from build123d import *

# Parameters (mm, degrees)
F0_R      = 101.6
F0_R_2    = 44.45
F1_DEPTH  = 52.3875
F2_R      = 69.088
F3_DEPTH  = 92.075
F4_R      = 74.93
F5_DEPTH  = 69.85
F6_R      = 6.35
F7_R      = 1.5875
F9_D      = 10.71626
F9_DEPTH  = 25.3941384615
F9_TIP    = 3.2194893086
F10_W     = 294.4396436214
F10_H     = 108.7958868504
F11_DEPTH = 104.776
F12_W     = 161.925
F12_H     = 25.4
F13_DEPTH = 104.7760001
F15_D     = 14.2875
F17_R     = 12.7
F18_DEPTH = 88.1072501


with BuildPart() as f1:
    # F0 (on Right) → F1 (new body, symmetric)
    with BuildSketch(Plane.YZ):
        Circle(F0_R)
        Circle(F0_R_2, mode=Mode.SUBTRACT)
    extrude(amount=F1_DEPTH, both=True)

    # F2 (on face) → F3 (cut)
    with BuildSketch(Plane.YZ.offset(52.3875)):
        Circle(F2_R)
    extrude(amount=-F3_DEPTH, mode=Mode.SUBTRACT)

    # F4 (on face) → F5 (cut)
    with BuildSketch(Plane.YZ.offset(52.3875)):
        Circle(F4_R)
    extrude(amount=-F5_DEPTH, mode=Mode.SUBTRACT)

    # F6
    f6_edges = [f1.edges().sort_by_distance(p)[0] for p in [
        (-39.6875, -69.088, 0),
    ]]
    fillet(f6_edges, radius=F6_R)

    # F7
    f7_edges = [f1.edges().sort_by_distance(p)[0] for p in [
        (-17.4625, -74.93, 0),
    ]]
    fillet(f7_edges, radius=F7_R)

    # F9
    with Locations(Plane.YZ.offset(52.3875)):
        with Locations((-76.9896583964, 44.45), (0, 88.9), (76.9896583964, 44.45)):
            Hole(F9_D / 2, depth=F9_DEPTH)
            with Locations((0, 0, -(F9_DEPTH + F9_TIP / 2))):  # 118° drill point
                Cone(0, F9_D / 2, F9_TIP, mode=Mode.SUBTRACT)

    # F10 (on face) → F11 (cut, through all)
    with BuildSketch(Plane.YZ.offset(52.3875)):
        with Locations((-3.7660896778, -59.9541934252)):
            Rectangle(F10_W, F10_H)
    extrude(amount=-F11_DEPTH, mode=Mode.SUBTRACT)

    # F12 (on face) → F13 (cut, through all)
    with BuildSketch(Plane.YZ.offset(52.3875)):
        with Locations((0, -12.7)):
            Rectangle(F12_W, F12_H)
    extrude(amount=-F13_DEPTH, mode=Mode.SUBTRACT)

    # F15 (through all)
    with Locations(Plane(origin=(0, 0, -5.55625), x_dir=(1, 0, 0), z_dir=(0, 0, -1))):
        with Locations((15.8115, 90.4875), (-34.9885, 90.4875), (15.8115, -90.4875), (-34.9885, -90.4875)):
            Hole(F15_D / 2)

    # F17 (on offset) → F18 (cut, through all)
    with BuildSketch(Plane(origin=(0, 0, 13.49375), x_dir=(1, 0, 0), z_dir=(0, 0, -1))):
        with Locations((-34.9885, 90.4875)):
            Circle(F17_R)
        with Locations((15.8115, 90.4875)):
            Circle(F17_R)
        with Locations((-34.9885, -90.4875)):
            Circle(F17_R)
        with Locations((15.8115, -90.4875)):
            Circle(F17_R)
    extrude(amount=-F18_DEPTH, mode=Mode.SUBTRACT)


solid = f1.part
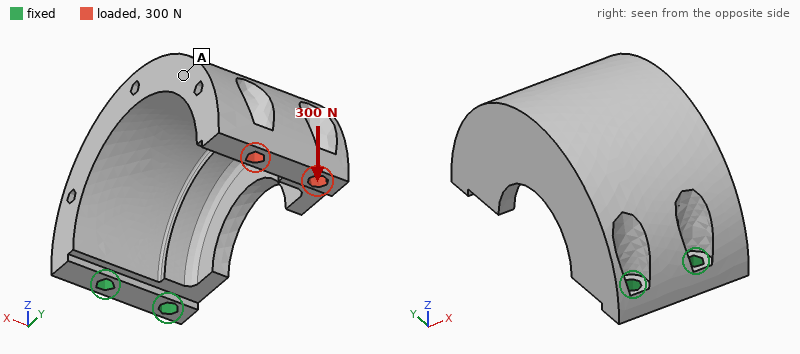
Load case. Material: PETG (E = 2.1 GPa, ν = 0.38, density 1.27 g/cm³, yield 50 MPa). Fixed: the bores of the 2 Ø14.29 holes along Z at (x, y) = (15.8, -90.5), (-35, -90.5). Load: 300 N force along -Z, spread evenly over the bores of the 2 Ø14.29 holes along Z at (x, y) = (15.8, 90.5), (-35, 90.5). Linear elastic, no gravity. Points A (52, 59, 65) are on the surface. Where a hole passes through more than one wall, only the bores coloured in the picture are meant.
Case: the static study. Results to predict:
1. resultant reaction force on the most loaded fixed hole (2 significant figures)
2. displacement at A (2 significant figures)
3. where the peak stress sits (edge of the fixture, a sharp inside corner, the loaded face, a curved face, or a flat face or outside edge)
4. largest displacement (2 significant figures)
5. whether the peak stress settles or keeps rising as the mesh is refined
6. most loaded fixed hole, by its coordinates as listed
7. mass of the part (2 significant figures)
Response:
230 N
2.0 mm
edge of the fixture
2.8 mm
keeps rising
(-35, -90.5)
1.0 kg
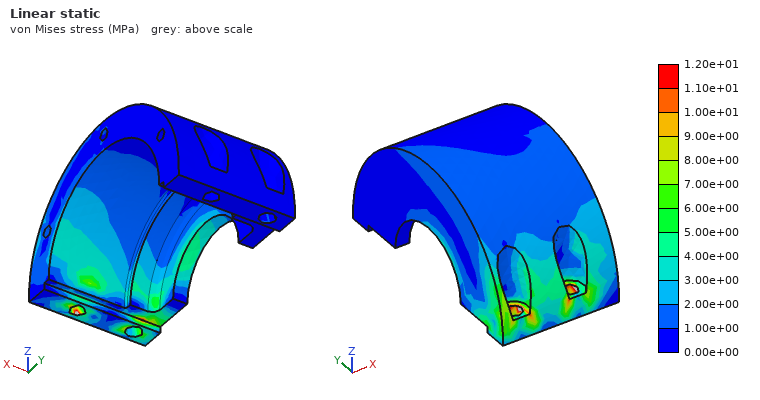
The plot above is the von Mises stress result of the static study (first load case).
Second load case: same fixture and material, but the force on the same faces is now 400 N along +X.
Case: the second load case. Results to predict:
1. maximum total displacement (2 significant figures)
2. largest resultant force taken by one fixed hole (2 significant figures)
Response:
2.9 mm
990 N
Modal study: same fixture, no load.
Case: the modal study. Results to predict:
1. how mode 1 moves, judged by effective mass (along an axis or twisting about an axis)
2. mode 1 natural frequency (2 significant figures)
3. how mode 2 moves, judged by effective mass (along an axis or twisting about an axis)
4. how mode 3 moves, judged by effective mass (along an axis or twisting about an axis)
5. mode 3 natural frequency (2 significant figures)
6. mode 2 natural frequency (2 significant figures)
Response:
along Z
88 Hz
along X
along Y
330 Hz
130 Hz
